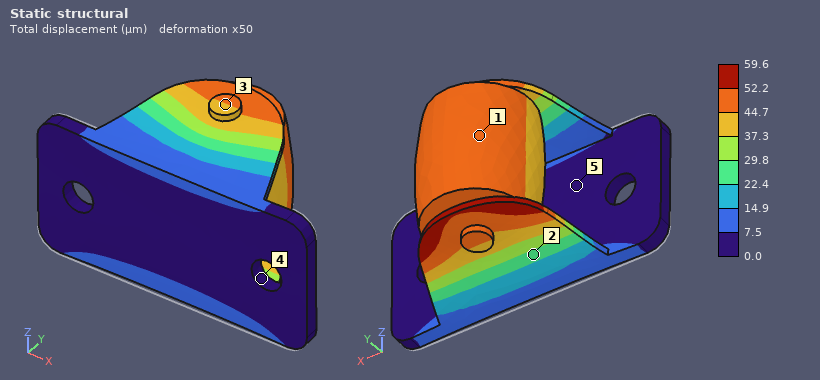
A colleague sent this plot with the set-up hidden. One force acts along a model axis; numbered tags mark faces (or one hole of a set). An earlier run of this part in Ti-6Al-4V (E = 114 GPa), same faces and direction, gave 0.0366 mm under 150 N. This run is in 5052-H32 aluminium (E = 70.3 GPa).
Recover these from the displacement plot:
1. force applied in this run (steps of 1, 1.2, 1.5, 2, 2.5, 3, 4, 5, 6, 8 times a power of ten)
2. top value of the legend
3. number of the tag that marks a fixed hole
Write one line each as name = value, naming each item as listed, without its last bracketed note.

force applied in this run = 150 N
top value of the legend = 59.6 µm
number of the tag that marks a fixed hole = 4
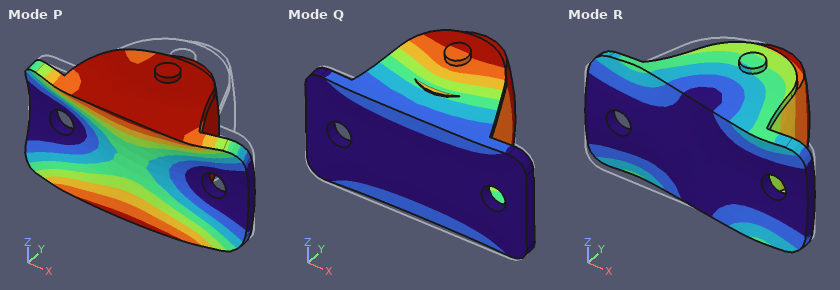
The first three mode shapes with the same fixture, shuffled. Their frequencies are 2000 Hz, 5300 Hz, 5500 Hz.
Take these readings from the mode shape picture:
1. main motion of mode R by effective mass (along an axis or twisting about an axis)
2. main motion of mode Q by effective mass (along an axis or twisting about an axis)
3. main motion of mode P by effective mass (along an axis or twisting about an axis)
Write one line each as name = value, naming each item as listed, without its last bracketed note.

main motion of mode R by effective mass = along X
main motion of mode Q by effective mass = along Z
main motion of mode P by effective mass = along Y
